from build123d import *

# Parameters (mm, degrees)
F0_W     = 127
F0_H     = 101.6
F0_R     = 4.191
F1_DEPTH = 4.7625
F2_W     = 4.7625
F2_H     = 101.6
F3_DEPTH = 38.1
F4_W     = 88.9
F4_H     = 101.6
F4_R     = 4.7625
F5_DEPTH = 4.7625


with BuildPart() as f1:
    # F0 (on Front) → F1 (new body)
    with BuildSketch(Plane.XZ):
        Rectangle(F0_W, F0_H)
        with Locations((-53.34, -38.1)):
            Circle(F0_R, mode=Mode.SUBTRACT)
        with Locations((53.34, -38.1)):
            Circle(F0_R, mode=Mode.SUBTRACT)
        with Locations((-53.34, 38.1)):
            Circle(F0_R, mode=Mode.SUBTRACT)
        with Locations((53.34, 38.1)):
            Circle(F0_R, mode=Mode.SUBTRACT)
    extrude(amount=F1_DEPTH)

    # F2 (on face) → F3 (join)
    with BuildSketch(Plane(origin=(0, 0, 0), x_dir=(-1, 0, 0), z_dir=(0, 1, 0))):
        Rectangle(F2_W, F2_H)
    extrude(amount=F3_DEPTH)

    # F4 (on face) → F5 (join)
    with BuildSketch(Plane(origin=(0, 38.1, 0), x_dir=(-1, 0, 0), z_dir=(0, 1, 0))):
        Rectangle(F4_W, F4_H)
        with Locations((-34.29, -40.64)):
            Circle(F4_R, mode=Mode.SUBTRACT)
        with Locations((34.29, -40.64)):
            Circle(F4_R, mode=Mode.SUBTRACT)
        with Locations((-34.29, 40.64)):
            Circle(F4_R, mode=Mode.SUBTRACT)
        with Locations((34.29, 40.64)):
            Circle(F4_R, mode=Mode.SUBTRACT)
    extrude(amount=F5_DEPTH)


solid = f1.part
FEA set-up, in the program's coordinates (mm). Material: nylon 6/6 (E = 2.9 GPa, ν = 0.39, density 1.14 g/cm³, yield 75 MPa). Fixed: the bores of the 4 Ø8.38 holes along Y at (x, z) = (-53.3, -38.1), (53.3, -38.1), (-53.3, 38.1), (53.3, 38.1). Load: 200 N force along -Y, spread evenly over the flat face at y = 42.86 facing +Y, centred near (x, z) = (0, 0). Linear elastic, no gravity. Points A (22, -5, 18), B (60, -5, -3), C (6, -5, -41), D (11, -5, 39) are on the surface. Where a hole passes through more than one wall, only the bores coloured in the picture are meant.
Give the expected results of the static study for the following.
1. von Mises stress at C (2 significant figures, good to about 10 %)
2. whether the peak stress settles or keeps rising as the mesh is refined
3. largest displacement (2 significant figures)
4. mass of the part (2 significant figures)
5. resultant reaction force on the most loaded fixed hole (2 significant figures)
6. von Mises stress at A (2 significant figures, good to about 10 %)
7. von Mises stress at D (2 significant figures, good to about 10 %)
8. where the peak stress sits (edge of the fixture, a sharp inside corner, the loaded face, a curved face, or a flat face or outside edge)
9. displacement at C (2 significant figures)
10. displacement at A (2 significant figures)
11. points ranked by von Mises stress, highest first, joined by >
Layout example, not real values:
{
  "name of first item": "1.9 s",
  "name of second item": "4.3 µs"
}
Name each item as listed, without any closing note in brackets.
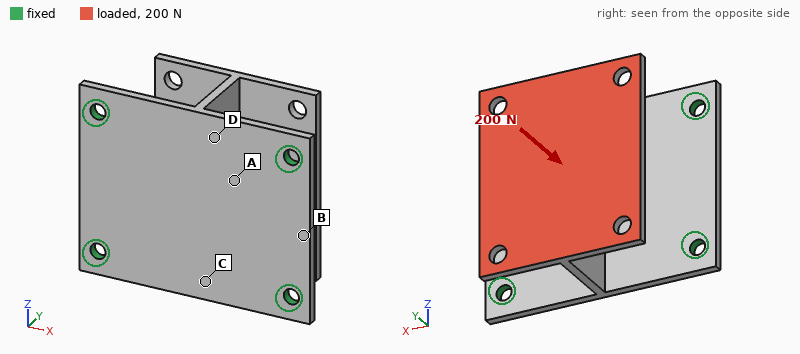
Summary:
{
  "von Mises stress at C": "5.7 MPa",
  "whether the peak stress settles or keeps rising as the mesh is refined": "keeps rising",
  "largest displacement": "0.83 mm",
  "mass of the part": "140 g",
  "resultant reaction force on the most loaded fixed hole": "50 N",
  "von Mises stress at A": "1.8 MPa",
  "von Mises stress at D": "4.3 MPa",
  "where the peak stress sits": "edge of the fixture",
  "displacement at C": "0.47 mm",
  "displacement at A": "0.34 mm",
  "points ranked by von Mises stress, highest first, joined by >": "C > D > A > B"
}
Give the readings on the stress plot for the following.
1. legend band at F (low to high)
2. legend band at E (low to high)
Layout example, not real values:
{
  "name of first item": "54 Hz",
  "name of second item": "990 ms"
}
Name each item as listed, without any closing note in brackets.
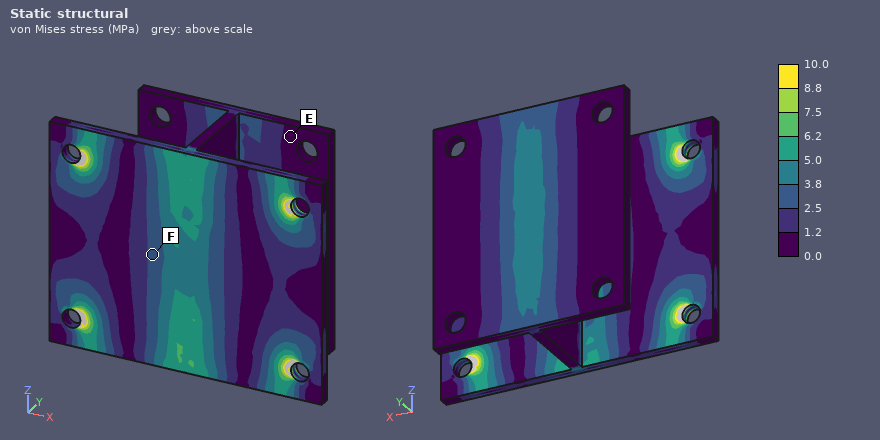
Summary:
{
  "legend band at F": "2.5 to 3.8 MPa",
  "legend band at E": "0.0 to 1.2 MPa"
}
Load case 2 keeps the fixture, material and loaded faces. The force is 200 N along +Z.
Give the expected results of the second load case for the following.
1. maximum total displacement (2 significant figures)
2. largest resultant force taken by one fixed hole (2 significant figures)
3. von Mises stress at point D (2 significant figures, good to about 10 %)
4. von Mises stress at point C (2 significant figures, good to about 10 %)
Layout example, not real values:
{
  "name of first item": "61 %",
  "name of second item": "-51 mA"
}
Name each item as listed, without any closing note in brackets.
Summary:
{
  "maximum total displacement": "1.0 mm",
  "largest resultant force taken by one fixed hole": "86 N",
  "von Mises stress at point D": "5.6 MPa",
  "von Mises stress at point C": "7.6 MPa"
}
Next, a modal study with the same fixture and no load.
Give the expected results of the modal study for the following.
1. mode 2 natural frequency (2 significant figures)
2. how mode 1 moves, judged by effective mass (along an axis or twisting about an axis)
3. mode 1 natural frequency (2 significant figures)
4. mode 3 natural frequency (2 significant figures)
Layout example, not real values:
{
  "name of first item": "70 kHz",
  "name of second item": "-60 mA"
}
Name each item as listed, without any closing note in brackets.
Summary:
{
  "mode 2 natural frequency": "290 Hz",
  "how mode 1 moves, judged by effective mass": "along X",
  "mode 1 natural frequency": "160 Hz",
  "mode 3 natural frequency": "300 Hz"
}
